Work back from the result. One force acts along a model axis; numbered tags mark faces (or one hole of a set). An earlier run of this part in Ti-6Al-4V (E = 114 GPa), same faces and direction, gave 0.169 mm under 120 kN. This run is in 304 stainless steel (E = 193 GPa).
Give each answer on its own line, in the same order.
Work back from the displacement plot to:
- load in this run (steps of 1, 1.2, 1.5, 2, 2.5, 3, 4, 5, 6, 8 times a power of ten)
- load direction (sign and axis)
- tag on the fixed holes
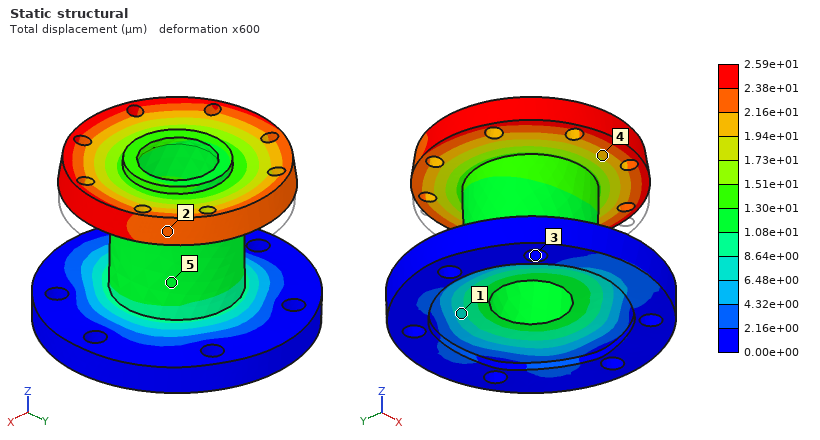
30 kN
+Z
3
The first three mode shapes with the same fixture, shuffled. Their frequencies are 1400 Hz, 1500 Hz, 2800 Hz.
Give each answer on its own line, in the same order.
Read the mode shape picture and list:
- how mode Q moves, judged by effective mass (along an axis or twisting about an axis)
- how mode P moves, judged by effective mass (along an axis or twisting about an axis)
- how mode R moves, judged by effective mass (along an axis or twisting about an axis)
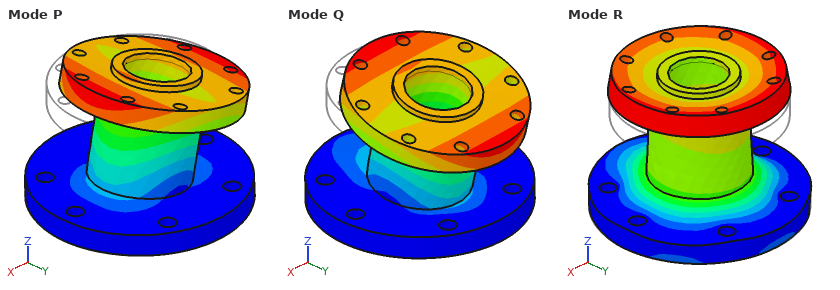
along Y
along X
along Z
